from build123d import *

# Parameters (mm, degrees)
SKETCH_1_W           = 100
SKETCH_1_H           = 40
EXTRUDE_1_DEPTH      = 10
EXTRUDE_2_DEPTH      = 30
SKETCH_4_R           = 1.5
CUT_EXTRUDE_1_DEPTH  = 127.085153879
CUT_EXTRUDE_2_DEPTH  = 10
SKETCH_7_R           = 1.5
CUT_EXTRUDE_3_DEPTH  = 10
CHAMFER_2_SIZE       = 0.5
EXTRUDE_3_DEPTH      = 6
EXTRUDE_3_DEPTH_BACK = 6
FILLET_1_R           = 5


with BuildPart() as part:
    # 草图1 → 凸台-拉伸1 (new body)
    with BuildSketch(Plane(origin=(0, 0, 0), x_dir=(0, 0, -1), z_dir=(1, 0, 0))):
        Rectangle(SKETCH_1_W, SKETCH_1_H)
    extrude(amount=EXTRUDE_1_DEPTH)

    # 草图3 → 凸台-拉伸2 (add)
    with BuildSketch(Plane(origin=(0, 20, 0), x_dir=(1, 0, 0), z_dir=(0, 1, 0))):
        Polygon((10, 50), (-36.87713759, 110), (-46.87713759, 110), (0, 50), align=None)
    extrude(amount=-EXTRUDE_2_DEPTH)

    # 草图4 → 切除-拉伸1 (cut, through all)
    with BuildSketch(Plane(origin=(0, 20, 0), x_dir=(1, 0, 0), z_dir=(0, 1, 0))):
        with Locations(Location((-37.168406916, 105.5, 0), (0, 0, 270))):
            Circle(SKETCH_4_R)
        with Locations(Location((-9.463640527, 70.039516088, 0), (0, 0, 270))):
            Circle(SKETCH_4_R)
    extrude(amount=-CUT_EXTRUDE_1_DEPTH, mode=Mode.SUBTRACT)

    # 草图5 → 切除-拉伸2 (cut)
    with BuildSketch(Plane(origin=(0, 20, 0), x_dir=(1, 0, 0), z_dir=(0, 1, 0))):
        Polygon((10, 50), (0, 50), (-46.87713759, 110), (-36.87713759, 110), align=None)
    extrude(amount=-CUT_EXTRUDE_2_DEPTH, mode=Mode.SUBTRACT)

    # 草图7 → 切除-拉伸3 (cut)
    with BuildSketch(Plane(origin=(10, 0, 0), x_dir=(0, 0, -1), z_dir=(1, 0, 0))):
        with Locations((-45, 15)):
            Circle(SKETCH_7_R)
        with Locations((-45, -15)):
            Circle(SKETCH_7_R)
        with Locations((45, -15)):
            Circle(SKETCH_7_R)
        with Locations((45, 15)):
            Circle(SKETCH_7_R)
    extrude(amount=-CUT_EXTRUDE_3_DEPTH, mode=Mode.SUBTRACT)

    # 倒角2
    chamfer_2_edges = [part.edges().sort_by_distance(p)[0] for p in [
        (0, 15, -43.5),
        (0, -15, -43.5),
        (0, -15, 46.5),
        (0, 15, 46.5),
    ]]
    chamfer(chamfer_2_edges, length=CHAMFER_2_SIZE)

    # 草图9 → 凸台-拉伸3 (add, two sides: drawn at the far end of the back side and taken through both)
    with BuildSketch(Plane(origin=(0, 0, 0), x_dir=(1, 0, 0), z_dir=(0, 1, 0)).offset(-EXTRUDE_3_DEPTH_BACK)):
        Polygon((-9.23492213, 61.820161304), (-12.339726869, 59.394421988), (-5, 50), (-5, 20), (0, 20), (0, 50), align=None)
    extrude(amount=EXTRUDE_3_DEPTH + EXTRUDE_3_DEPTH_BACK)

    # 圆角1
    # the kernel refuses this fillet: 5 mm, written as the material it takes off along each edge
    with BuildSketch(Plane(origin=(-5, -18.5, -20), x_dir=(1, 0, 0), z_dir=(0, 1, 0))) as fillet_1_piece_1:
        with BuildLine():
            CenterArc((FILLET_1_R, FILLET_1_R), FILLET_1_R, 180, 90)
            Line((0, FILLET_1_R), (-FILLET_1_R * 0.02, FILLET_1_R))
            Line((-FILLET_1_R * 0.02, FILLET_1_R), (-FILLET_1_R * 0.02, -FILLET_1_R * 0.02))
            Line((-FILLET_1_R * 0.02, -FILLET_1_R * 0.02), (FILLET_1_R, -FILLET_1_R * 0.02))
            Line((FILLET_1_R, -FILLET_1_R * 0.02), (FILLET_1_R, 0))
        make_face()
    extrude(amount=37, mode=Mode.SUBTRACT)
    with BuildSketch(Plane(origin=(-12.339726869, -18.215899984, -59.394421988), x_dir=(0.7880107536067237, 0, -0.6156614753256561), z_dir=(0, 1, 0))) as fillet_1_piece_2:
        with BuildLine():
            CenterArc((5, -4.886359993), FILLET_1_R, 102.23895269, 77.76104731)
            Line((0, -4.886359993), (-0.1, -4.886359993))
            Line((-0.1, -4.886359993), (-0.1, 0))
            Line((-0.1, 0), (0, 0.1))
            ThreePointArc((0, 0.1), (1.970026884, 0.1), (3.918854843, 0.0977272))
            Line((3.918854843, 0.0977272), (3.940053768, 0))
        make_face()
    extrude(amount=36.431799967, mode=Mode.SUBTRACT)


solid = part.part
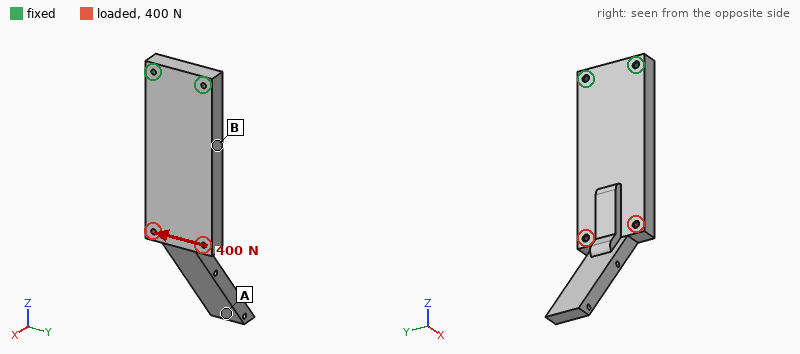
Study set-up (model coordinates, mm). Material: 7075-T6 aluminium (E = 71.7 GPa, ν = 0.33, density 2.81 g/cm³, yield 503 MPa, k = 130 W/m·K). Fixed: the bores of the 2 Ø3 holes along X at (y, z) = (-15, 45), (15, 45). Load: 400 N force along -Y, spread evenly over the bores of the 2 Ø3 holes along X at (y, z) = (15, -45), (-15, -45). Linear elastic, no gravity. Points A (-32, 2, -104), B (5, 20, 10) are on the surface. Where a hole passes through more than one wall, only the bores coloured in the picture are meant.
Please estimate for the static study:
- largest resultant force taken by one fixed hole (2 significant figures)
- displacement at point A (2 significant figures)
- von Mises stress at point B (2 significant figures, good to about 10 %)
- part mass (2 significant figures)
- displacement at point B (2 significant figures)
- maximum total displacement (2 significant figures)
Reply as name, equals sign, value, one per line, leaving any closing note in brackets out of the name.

largest resultant force taken by one fixed hole = 1.2 kN
displacement at point A = 55 µm
von Mises stress at point B = 8.3 MPa
part mass = 150 g
displacement at point B = 9.3 µm
maximum total displacement = 57 µm
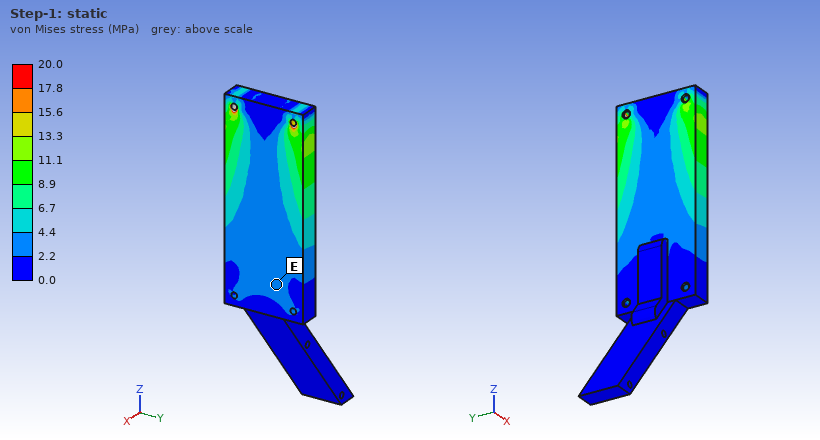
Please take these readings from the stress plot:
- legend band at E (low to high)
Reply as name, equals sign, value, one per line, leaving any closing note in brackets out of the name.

legend band at E = 2.2 to 4.4 MPa
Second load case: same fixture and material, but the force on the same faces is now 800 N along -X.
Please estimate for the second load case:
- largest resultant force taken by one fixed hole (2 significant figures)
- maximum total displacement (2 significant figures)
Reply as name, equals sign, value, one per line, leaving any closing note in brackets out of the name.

largest resultant force taken by one fixed hole = 400 N
maximum total displacement = 2.1 mm
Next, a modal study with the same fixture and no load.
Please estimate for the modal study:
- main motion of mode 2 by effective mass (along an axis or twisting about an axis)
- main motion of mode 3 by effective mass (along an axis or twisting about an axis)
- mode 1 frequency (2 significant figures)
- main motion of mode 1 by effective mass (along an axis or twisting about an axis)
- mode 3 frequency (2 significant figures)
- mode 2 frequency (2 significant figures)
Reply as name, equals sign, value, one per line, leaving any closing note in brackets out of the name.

main motion of mode 2 by effective mass = along Y
main motion of mode 3 by effective mass = along X
mode 1 frequency = 400 Hz
main motion of mode 1 by effective mass = along X
mode 3 frequency = 1600 Hz
mode 2 frequency = 1200 Hz
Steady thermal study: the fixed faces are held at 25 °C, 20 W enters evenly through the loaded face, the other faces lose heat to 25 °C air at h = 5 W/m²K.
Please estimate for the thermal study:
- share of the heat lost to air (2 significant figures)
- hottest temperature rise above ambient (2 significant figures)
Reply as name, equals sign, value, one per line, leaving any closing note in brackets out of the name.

share of the heat lost to air = 8.4 %
hottest temperature rise above ambient = 36 K
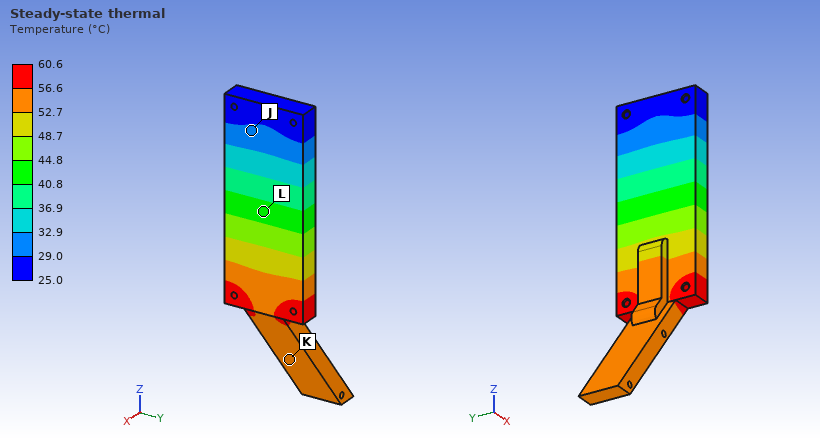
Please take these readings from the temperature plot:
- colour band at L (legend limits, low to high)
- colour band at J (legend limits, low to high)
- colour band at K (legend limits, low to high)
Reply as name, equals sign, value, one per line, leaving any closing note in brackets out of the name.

colour band at L = 40.8 to 44.8 °C
colour band at J = 29.0 to 32.9 °C
colour band at K = 52.7 to 56.6 °C
